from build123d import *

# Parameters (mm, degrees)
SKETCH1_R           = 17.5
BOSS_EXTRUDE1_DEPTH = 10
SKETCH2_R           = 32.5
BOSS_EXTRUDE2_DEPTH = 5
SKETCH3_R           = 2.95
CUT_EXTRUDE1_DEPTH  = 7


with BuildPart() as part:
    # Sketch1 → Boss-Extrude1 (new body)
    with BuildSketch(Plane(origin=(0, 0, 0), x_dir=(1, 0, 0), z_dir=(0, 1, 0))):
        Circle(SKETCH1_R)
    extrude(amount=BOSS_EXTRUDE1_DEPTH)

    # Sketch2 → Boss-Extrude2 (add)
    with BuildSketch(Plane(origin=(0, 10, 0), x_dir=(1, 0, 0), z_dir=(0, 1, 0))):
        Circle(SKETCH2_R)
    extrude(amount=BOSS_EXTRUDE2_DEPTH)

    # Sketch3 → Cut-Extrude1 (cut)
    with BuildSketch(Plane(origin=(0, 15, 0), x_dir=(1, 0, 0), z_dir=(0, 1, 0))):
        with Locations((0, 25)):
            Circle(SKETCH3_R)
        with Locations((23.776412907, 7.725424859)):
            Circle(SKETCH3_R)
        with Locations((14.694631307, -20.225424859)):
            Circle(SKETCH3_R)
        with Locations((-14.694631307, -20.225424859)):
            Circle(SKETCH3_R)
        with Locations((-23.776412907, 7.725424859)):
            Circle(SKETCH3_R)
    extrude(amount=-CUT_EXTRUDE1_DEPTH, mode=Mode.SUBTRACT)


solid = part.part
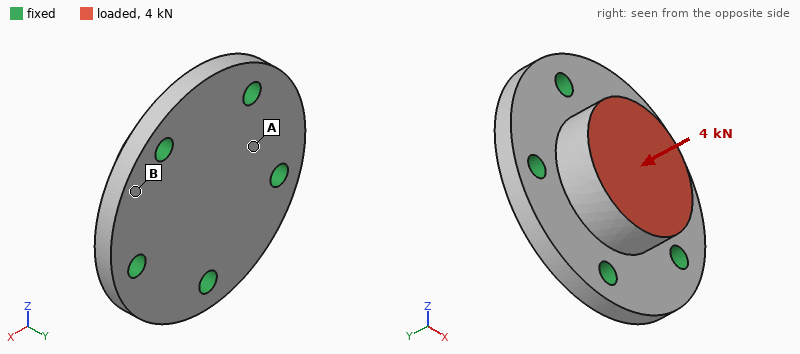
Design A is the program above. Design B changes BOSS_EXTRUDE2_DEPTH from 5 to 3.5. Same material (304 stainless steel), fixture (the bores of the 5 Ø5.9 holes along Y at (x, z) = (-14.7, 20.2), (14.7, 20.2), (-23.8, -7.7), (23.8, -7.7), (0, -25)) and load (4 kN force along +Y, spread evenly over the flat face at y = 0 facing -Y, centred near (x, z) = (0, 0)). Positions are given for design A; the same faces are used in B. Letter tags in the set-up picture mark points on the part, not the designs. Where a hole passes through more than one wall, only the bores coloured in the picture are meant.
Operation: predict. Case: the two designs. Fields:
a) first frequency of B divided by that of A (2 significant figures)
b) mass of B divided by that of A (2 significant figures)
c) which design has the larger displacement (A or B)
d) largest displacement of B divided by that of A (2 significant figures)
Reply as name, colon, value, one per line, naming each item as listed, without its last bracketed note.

first frequency of B divided by that of A: 0.79
mass of B divided by that of A: 0.81
which design has the larger displacement: B
largest displacement of B divided by that of A: 1.7
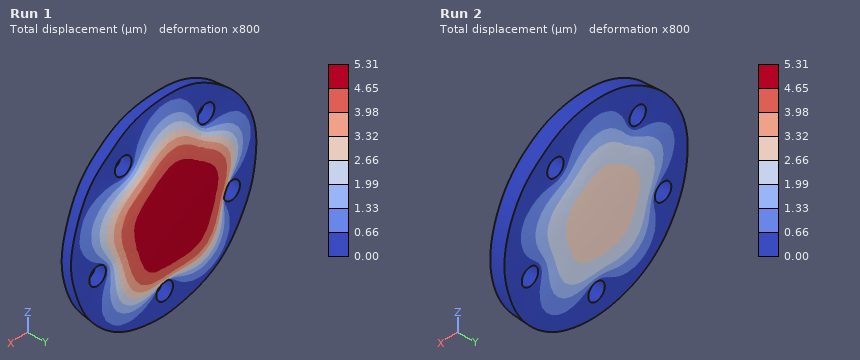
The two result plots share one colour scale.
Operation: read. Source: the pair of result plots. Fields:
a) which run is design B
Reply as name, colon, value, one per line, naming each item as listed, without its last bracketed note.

which run is design B: Run 1
